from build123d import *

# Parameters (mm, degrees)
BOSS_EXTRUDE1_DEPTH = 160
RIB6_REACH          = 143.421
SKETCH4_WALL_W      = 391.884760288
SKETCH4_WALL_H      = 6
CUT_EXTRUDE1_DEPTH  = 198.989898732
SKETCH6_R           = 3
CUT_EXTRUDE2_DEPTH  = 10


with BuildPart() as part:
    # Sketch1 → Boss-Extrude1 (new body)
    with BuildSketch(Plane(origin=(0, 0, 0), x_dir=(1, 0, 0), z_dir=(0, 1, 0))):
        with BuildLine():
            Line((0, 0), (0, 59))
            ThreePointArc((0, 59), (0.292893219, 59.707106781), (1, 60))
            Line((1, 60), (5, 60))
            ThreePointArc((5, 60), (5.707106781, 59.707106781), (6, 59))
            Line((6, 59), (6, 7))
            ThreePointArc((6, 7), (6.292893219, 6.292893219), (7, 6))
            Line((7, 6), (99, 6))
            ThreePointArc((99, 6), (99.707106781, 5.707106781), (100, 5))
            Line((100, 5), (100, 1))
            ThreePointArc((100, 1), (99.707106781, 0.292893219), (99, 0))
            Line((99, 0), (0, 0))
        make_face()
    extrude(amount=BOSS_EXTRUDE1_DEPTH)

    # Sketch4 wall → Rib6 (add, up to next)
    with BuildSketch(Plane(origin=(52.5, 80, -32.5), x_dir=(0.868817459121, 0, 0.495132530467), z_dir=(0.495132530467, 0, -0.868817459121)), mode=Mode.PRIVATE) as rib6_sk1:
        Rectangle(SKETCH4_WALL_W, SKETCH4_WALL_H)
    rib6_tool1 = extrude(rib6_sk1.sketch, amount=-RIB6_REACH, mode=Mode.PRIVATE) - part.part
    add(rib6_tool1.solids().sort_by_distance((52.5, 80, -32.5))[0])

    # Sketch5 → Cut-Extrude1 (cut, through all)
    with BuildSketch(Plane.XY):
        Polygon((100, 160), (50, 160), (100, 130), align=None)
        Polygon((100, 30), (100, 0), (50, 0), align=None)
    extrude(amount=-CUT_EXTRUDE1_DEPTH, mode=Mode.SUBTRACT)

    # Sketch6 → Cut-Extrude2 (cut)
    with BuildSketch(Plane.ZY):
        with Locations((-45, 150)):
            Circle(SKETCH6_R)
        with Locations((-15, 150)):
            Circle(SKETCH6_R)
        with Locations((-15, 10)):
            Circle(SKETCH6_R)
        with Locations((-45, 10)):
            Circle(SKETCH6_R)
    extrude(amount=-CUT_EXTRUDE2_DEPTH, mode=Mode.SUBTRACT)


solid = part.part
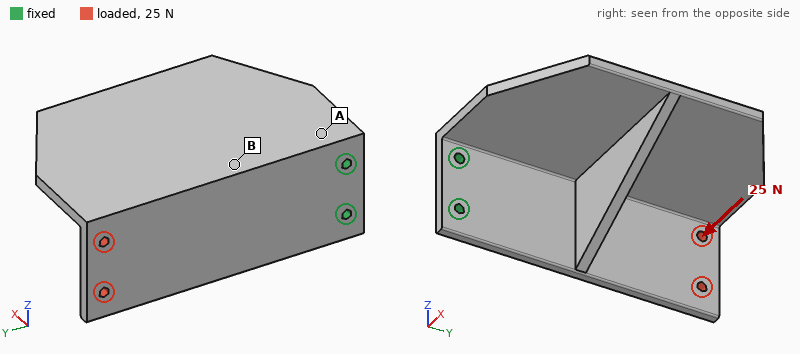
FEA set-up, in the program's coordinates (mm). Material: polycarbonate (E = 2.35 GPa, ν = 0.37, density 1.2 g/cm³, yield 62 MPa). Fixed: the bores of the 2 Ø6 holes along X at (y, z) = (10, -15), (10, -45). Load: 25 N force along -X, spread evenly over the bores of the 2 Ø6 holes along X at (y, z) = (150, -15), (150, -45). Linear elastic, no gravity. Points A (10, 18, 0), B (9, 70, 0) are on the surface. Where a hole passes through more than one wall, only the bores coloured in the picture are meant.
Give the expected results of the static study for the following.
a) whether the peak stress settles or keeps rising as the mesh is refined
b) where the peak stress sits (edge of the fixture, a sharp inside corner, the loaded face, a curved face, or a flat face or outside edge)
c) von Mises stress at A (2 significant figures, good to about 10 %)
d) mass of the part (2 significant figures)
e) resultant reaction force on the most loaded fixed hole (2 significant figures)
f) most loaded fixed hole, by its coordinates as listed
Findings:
keeps rising
edge of the fixture
1.3 MPa
180 g
18 N
(10, -15)
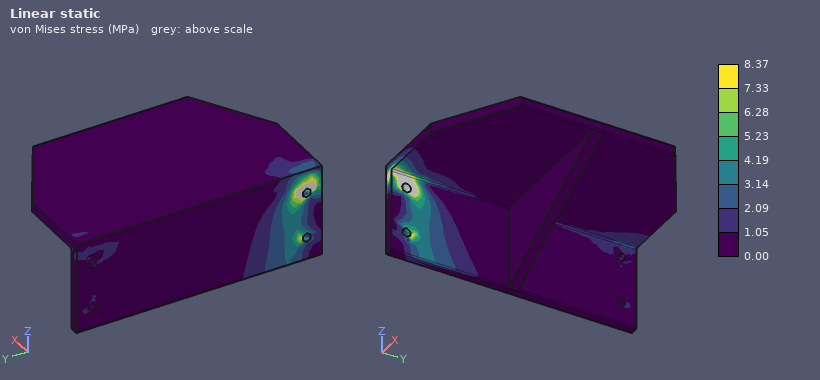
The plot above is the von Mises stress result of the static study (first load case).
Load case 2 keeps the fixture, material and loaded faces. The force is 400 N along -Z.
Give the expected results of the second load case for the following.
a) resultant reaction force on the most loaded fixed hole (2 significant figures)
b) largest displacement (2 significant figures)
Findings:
1.6 kN
2.0 mm
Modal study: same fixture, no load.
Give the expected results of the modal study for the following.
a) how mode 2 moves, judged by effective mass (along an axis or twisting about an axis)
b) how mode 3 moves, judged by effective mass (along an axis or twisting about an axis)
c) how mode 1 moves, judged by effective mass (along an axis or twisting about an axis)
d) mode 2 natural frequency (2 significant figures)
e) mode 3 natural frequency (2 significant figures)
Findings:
along Z
twisting about X
along X
100 Hz
290 Hz
